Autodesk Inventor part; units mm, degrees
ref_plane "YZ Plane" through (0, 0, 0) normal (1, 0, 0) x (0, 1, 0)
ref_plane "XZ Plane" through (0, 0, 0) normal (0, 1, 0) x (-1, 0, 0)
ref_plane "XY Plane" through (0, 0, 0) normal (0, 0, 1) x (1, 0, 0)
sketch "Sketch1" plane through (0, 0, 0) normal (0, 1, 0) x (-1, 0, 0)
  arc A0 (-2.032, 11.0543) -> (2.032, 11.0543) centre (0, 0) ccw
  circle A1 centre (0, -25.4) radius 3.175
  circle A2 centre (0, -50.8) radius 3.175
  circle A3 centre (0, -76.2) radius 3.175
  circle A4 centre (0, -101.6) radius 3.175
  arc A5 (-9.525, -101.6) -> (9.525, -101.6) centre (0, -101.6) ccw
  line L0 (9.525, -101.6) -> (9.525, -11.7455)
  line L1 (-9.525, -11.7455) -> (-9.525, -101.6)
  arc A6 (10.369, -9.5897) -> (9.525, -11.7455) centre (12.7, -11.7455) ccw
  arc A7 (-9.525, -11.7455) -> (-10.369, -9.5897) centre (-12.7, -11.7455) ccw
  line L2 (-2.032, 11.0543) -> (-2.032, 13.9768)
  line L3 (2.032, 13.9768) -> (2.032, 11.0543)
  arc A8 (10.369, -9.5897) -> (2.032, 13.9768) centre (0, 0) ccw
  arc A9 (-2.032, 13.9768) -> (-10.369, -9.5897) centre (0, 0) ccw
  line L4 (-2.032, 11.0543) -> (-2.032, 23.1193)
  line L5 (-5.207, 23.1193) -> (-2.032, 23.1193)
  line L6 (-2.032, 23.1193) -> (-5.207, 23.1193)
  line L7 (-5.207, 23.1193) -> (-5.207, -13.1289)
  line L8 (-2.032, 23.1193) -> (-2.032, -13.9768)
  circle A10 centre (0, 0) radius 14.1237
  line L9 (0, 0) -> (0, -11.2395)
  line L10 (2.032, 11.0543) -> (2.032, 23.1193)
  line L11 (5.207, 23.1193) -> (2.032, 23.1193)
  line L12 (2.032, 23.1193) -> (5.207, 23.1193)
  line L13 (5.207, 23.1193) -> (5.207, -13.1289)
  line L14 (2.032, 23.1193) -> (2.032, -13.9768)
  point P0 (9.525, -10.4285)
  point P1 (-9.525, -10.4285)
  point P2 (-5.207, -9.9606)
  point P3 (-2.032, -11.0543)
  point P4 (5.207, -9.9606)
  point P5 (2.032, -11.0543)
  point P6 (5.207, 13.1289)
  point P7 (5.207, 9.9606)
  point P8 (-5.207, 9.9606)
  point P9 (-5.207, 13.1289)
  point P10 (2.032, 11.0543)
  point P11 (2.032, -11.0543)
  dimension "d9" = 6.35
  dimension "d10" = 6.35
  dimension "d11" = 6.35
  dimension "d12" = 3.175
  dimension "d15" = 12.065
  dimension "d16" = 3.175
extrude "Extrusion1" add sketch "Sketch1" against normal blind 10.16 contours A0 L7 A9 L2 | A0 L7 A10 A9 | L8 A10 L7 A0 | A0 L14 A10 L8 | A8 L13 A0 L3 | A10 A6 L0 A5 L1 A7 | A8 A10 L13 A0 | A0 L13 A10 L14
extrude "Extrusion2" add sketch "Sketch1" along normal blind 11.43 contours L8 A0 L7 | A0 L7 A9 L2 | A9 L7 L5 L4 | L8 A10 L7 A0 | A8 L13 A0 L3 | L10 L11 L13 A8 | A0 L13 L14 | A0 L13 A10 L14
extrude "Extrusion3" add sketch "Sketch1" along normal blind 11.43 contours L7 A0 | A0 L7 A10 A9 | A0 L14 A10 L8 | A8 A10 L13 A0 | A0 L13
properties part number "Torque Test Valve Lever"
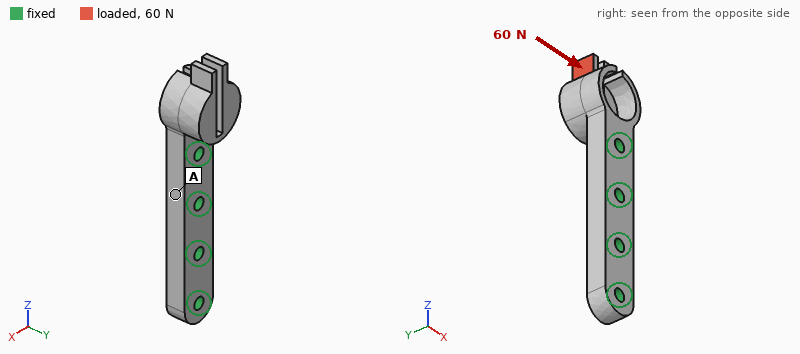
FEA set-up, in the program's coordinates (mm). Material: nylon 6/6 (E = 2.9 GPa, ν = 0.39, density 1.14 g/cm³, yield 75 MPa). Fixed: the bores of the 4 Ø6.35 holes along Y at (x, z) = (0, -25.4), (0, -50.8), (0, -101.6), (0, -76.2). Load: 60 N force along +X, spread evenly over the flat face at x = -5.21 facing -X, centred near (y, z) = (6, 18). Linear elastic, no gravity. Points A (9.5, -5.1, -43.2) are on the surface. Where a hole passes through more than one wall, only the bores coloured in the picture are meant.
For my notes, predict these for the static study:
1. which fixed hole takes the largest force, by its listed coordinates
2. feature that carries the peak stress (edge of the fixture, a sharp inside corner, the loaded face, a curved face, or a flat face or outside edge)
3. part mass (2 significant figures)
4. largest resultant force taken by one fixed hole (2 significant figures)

(0, -25.4)
a curved face
30 g
110 N
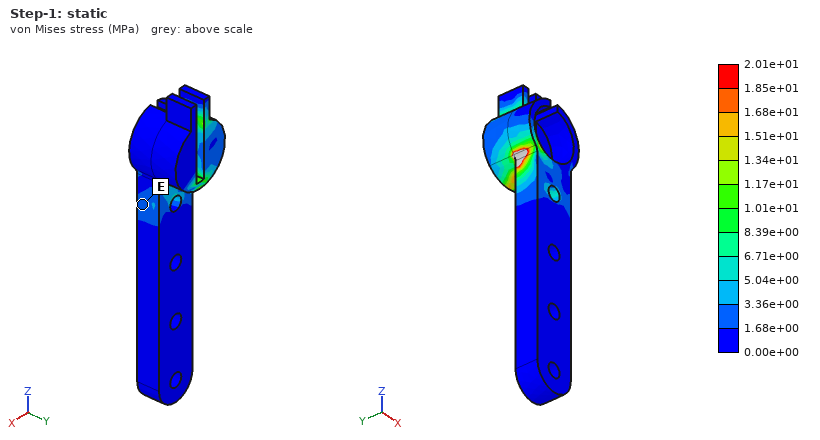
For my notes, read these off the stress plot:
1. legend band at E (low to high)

1.68e+00 to 3.36e+00 MPa
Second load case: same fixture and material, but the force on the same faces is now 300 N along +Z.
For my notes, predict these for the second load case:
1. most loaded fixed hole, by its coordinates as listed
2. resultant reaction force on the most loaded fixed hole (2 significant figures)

(0, -25.4)
280 N
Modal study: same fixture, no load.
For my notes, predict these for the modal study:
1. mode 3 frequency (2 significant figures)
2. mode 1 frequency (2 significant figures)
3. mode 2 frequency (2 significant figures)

1200 Hz
880 Hz
900 Hz
